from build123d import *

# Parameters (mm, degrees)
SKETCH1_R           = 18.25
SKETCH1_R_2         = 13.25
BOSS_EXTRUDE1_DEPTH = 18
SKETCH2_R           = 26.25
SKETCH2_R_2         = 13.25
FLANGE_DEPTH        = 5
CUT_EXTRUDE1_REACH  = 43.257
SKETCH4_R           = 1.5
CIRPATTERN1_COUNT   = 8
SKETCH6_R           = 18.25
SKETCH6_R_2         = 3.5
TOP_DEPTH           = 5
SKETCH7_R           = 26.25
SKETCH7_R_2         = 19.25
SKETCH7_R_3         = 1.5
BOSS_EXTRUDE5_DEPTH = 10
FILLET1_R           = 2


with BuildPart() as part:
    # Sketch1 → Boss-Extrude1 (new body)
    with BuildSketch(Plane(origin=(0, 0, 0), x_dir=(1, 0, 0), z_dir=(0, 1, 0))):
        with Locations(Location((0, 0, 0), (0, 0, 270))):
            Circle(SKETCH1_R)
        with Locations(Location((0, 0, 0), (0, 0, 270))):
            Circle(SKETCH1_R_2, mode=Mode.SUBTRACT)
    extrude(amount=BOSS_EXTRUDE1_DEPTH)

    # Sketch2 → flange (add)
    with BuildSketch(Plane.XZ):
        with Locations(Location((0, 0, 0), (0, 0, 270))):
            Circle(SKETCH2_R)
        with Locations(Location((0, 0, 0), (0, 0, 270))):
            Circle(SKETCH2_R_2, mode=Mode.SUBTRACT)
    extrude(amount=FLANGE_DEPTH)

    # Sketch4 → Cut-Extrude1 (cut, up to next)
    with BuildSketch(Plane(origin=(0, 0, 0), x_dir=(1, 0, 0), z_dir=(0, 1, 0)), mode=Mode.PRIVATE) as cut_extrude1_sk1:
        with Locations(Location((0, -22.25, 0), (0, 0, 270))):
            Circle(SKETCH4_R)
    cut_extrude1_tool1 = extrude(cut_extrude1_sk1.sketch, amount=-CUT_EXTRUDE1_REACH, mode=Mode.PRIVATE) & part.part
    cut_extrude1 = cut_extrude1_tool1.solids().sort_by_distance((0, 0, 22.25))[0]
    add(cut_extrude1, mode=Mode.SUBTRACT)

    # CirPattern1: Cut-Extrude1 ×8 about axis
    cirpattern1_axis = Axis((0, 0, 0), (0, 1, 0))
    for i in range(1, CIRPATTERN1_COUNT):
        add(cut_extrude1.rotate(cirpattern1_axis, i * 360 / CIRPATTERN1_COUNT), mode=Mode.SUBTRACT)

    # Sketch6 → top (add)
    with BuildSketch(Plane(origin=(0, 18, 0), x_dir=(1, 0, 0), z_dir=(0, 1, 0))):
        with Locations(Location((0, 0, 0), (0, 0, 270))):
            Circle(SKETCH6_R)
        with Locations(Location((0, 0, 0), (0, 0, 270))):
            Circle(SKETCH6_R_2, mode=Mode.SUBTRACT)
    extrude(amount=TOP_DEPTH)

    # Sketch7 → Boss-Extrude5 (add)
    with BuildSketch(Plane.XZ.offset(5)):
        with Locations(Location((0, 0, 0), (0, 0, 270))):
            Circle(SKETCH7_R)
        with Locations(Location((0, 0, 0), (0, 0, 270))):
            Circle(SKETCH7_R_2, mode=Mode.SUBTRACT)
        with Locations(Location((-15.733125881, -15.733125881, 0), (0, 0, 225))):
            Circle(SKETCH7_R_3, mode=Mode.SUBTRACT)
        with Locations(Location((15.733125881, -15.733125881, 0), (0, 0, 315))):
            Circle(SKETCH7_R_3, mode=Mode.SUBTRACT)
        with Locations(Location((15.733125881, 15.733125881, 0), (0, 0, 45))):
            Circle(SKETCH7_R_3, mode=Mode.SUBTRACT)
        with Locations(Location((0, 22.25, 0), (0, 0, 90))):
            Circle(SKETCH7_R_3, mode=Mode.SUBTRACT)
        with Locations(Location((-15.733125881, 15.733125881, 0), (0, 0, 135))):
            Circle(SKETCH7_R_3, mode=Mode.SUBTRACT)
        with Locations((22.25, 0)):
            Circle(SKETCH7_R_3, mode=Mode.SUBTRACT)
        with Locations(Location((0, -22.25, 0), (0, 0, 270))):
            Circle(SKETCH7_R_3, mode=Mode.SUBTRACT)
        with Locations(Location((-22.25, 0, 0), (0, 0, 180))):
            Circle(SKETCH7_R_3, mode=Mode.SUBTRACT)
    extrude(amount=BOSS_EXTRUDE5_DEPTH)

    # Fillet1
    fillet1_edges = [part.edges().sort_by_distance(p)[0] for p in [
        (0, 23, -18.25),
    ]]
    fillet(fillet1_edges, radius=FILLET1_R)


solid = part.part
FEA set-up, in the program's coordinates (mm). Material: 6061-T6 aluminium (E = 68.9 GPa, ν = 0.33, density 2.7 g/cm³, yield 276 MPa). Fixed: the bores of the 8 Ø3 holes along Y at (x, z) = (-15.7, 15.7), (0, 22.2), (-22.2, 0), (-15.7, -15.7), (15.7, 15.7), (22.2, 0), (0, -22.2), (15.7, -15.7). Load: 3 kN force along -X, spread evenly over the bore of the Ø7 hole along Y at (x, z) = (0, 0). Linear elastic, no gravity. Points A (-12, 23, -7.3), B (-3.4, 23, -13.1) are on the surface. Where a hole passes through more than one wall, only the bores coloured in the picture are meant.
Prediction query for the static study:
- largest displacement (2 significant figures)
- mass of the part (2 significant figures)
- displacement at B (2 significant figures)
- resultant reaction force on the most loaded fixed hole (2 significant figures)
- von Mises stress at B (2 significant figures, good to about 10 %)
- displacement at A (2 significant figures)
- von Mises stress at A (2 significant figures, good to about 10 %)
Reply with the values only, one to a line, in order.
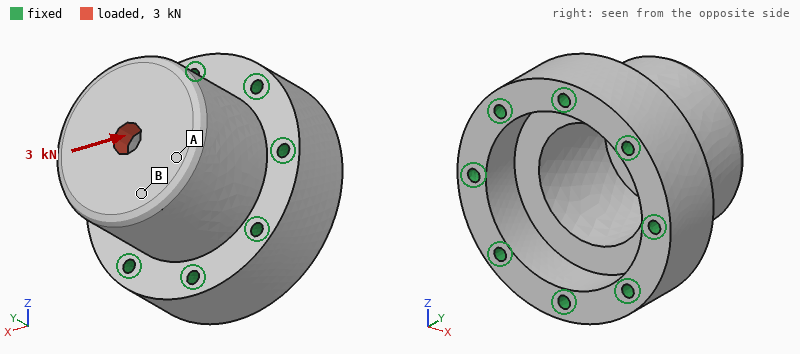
20 µm
84 g
15 µm
1.0 kN
4.7 MPa
18 µm
16 MPa
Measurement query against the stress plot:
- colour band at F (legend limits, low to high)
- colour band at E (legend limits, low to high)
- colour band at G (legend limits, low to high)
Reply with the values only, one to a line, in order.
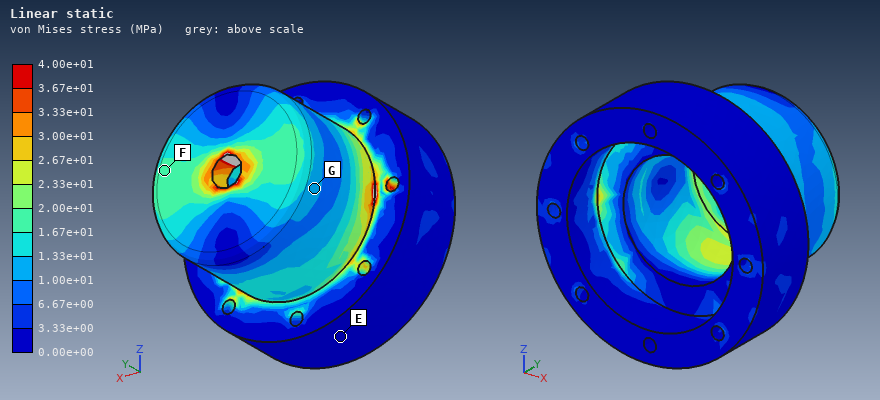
1.67e+01 to 2.00e+01 MPa
0.00e+00 to 3.33e+00 MPa
1.00e+01 to 1.33e+01 MPa
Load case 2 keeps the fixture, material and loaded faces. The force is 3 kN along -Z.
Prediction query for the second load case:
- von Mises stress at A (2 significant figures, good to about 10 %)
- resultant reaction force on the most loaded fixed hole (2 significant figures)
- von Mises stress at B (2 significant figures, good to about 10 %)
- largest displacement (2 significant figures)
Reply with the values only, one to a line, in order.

9.4 MPa
1.0 kN
18 MPa
20 µm
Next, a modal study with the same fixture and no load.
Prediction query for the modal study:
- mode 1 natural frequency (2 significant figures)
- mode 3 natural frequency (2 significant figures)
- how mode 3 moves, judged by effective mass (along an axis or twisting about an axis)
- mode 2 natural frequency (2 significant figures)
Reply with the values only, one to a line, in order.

15 kHz
26 kHz
along Y
15 kHz
